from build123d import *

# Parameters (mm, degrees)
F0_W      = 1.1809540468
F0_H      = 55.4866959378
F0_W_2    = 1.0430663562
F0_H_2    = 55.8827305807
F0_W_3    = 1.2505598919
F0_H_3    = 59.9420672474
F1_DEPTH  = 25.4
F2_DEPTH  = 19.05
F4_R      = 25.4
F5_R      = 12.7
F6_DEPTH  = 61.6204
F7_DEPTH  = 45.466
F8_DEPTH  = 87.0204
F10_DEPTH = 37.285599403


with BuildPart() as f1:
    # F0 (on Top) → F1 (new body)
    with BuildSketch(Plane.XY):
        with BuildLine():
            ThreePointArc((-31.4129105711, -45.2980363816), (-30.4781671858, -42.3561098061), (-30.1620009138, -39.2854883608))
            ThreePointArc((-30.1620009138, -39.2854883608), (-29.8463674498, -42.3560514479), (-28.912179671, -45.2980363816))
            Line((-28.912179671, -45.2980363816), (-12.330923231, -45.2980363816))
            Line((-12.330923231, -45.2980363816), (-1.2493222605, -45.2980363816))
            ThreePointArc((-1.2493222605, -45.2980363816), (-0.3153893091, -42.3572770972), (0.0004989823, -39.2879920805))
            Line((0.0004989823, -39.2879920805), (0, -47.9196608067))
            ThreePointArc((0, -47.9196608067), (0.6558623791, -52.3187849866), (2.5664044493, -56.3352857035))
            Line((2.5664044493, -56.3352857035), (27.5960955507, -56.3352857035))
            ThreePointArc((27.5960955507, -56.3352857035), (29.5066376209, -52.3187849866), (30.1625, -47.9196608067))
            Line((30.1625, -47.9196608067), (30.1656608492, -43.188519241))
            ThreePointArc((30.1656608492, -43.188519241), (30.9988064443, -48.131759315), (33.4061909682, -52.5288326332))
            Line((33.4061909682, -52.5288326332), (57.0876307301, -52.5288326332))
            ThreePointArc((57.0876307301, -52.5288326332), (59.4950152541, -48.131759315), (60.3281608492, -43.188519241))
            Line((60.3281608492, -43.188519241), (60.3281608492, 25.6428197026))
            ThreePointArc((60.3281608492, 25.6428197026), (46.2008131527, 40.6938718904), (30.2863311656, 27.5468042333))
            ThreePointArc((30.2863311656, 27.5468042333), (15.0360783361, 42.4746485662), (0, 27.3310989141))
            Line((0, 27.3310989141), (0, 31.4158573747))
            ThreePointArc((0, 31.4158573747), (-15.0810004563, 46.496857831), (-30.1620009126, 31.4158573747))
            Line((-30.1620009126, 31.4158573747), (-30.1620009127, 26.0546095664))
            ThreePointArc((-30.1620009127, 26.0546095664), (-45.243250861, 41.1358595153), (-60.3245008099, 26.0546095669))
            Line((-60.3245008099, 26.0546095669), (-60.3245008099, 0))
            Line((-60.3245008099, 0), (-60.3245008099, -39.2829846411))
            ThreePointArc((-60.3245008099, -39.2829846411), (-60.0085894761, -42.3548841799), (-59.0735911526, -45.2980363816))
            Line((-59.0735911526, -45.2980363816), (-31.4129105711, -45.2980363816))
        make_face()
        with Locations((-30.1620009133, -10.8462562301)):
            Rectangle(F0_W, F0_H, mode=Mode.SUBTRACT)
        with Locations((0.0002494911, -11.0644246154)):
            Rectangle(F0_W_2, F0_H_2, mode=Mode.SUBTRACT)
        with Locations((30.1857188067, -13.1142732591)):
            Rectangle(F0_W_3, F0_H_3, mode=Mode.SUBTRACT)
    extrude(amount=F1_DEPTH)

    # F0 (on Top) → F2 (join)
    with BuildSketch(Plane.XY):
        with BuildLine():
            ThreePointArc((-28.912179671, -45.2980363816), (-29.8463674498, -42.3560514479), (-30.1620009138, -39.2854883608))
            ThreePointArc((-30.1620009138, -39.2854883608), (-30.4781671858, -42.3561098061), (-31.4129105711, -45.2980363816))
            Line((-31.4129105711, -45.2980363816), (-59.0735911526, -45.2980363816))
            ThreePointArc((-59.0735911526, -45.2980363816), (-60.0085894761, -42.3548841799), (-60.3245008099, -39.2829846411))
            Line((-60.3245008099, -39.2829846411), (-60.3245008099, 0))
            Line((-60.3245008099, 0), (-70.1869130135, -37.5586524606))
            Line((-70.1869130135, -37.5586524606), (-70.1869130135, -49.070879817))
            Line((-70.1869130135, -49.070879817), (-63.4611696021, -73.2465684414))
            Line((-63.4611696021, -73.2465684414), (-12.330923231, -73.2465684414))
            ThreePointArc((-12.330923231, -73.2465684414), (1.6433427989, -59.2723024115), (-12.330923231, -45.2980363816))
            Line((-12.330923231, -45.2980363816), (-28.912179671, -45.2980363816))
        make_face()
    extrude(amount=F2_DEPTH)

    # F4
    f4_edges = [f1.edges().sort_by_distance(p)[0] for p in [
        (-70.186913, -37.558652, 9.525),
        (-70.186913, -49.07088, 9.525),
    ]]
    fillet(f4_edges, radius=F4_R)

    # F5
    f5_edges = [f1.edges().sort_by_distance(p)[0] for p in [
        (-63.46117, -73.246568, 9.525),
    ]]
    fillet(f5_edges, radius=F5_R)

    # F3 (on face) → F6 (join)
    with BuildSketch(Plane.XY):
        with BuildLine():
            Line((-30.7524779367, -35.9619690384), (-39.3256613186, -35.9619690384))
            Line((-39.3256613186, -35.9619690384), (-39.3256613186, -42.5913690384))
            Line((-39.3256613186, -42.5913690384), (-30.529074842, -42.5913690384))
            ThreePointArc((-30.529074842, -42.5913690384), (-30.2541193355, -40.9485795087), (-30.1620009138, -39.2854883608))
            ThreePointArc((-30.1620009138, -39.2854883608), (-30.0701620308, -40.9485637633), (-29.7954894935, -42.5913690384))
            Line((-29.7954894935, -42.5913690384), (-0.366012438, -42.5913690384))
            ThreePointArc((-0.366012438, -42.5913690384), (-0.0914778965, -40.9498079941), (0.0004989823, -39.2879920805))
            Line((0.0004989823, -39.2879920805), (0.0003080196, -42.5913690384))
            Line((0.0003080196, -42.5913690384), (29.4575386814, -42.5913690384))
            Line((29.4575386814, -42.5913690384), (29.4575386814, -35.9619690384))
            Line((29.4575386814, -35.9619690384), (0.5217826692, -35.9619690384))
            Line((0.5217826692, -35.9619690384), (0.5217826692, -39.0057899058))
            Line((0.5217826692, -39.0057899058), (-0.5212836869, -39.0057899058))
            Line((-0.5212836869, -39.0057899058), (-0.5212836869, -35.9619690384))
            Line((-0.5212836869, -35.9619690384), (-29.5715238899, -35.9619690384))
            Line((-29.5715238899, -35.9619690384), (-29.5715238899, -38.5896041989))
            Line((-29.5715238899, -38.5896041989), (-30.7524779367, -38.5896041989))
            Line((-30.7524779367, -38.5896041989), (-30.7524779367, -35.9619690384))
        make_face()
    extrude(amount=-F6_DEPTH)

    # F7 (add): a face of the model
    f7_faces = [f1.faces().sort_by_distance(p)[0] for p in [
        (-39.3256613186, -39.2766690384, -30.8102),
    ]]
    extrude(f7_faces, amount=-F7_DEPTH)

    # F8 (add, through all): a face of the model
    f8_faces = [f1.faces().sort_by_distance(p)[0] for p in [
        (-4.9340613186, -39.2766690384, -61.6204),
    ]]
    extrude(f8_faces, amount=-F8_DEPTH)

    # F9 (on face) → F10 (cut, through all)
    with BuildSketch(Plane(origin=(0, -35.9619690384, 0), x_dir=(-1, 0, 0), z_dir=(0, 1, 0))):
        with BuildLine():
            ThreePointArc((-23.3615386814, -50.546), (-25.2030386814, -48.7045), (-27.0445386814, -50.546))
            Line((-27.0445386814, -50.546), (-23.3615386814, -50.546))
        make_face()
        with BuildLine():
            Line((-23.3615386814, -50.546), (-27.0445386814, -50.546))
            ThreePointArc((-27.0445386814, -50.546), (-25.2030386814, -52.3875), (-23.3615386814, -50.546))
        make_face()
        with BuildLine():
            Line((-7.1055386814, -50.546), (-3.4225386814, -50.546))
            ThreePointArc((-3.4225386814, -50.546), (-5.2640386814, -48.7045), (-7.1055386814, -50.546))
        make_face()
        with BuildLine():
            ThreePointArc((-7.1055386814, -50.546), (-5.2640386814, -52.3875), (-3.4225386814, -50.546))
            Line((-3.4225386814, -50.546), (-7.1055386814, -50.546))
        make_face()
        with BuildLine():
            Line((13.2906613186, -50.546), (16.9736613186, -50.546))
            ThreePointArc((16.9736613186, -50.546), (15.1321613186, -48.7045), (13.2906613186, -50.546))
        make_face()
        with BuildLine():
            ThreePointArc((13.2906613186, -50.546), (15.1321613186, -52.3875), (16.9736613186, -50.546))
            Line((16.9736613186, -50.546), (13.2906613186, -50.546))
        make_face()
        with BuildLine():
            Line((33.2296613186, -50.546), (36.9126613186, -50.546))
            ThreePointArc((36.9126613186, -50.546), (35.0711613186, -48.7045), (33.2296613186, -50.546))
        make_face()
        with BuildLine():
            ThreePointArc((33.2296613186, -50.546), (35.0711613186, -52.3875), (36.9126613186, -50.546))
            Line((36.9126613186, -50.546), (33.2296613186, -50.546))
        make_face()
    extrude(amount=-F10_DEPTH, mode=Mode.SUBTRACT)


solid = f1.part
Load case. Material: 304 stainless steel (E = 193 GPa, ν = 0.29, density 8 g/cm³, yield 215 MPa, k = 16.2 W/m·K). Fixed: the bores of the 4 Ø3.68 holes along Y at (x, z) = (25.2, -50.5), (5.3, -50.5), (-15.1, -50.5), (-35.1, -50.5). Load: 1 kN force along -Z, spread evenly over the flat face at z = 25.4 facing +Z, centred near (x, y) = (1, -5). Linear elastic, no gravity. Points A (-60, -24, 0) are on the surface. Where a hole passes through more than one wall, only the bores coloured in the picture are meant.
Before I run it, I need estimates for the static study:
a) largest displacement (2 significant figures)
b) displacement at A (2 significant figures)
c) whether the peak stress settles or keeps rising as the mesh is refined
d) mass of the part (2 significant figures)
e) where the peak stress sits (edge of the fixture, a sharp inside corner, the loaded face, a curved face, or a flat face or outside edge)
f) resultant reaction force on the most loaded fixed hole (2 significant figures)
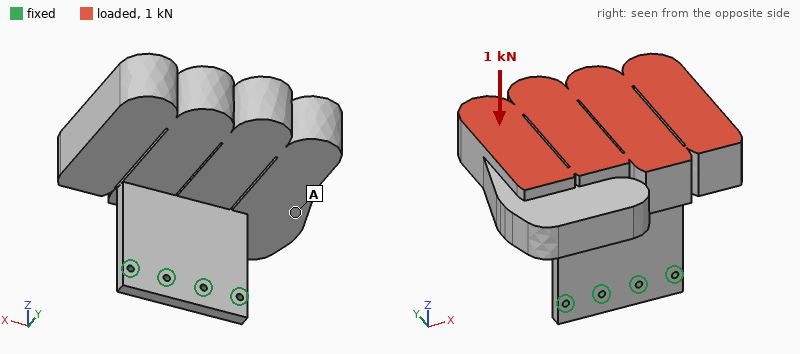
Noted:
0.54 mm
0.16 mm
keeps rising
2.7 kg
edge of the fixture
340 N
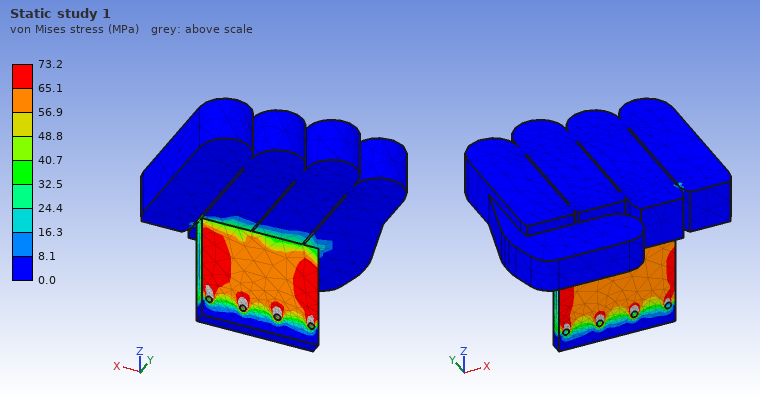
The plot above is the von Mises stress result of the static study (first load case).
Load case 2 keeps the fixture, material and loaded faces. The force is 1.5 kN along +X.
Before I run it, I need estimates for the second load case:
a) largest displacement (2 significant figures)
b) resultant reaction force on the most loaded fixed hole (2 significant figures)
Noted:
0.26 mm
1.9 kN
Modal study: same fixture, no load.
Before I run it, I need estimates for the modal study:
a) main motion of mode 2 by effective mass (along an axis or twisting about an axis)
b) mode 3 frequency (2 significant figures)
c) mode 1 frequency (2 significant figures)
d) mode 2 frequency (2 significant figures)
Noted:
along X
670 Hz
140 Hz
260 Hz
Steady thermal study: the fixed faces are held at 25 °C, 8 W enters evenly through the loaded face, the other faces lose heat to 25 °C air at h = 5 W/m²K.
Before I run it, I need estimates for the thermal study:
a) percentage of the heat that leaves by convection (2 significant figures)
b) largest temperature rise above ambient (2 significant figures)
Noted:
64 %
29 K
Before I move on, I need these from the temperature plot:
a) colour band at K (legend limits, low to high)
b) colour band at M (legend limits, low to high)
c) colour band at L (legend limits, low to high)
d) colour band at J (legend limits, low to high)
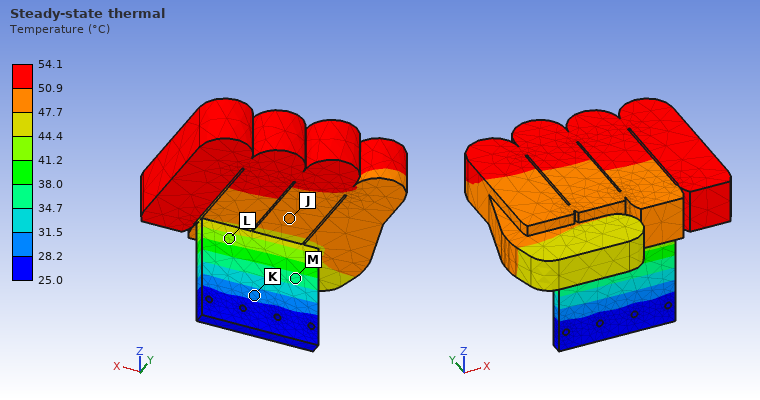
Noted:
28.2 to 31.5 °C
34.7 to 38.0 °C
41.2 to 44.4 °C
47.7 to 50.9 °C
